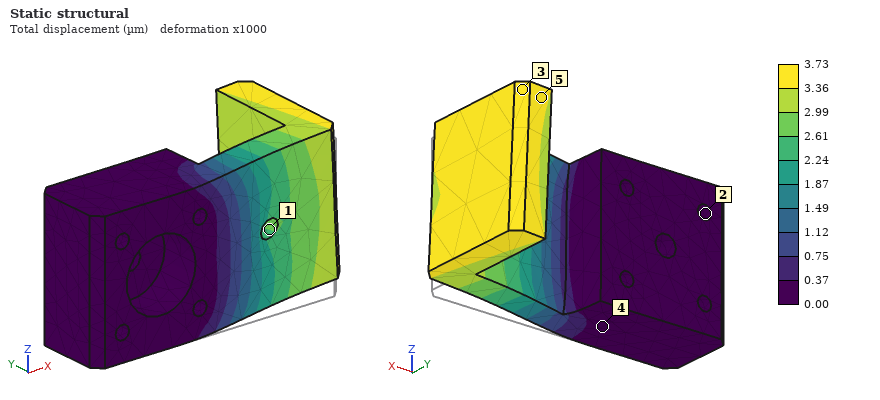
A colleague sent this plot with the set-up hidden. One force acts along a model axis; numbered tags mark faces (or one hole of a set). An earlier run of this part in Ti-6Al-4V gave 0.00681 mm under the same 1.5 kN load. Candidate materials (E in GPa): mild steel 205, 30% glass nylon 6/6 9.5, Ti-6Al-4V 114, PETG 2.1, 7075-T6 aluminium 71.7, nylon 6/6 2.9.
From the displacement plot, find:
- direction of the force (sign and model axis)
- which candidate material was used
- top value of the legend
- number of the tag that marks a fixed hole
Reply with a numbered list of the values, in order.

1. +Z
2. mild steel
3. 3.73 µm
4. 2
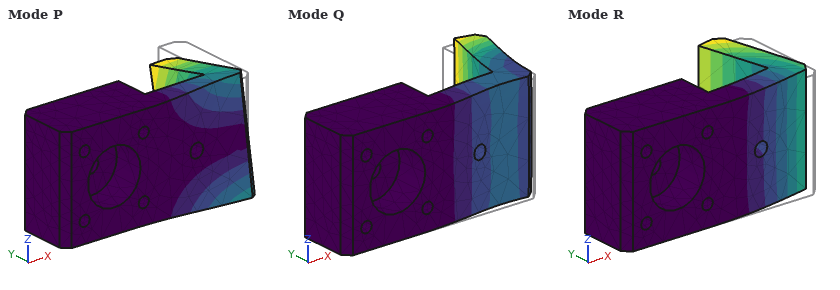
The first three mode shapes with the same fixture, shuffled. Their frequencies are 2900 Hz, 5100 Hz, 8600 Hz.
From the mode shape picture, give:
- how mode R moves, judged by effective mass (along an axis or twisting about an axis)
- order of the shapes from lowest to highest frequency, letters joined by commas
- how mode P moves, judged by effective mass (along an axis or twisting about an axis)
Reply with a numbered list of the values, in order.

1. along Y
2. R, P, Q
3. along Z
